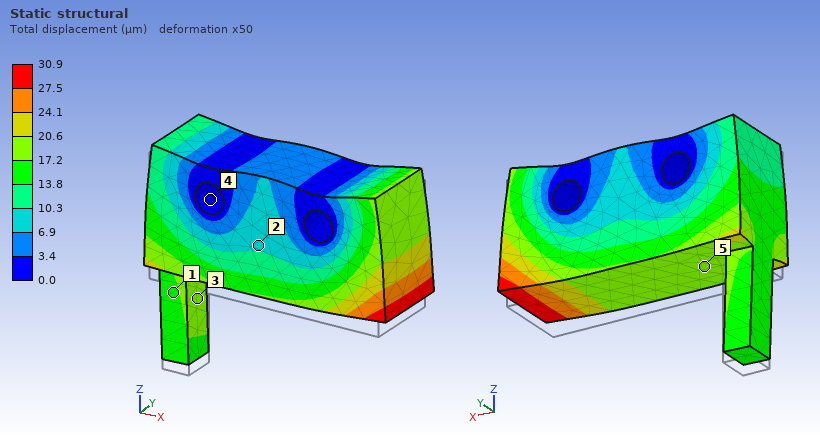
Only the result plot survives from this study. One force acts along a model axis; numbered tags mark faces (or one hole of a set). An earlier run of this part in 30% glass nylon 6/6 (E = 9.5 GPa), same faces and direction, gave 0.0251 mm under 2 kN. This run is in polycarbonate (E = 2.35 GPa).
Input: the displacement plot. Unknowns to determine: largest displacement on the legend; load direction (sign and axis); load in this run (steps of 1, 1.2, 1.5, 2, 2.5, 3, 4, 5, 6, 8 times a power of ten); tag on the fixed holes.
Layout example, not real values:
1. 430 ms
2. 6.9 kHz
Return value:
1. 30.9 µm
2. +Z
3. 600 N
4. 4
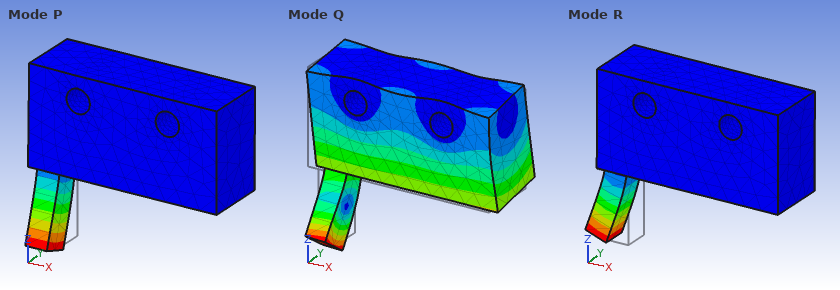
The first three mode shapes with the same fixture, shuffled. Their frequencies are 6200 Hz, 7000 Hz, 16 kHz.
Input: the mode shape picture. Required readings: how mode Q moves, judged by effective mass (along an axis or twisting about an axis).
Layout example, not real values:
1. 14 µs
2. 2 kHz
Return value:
1. along Y
